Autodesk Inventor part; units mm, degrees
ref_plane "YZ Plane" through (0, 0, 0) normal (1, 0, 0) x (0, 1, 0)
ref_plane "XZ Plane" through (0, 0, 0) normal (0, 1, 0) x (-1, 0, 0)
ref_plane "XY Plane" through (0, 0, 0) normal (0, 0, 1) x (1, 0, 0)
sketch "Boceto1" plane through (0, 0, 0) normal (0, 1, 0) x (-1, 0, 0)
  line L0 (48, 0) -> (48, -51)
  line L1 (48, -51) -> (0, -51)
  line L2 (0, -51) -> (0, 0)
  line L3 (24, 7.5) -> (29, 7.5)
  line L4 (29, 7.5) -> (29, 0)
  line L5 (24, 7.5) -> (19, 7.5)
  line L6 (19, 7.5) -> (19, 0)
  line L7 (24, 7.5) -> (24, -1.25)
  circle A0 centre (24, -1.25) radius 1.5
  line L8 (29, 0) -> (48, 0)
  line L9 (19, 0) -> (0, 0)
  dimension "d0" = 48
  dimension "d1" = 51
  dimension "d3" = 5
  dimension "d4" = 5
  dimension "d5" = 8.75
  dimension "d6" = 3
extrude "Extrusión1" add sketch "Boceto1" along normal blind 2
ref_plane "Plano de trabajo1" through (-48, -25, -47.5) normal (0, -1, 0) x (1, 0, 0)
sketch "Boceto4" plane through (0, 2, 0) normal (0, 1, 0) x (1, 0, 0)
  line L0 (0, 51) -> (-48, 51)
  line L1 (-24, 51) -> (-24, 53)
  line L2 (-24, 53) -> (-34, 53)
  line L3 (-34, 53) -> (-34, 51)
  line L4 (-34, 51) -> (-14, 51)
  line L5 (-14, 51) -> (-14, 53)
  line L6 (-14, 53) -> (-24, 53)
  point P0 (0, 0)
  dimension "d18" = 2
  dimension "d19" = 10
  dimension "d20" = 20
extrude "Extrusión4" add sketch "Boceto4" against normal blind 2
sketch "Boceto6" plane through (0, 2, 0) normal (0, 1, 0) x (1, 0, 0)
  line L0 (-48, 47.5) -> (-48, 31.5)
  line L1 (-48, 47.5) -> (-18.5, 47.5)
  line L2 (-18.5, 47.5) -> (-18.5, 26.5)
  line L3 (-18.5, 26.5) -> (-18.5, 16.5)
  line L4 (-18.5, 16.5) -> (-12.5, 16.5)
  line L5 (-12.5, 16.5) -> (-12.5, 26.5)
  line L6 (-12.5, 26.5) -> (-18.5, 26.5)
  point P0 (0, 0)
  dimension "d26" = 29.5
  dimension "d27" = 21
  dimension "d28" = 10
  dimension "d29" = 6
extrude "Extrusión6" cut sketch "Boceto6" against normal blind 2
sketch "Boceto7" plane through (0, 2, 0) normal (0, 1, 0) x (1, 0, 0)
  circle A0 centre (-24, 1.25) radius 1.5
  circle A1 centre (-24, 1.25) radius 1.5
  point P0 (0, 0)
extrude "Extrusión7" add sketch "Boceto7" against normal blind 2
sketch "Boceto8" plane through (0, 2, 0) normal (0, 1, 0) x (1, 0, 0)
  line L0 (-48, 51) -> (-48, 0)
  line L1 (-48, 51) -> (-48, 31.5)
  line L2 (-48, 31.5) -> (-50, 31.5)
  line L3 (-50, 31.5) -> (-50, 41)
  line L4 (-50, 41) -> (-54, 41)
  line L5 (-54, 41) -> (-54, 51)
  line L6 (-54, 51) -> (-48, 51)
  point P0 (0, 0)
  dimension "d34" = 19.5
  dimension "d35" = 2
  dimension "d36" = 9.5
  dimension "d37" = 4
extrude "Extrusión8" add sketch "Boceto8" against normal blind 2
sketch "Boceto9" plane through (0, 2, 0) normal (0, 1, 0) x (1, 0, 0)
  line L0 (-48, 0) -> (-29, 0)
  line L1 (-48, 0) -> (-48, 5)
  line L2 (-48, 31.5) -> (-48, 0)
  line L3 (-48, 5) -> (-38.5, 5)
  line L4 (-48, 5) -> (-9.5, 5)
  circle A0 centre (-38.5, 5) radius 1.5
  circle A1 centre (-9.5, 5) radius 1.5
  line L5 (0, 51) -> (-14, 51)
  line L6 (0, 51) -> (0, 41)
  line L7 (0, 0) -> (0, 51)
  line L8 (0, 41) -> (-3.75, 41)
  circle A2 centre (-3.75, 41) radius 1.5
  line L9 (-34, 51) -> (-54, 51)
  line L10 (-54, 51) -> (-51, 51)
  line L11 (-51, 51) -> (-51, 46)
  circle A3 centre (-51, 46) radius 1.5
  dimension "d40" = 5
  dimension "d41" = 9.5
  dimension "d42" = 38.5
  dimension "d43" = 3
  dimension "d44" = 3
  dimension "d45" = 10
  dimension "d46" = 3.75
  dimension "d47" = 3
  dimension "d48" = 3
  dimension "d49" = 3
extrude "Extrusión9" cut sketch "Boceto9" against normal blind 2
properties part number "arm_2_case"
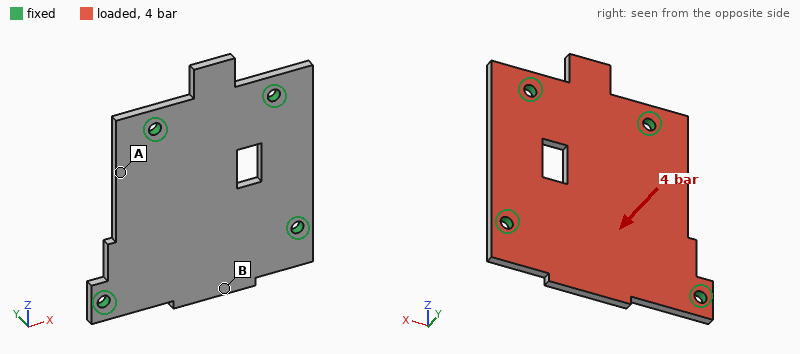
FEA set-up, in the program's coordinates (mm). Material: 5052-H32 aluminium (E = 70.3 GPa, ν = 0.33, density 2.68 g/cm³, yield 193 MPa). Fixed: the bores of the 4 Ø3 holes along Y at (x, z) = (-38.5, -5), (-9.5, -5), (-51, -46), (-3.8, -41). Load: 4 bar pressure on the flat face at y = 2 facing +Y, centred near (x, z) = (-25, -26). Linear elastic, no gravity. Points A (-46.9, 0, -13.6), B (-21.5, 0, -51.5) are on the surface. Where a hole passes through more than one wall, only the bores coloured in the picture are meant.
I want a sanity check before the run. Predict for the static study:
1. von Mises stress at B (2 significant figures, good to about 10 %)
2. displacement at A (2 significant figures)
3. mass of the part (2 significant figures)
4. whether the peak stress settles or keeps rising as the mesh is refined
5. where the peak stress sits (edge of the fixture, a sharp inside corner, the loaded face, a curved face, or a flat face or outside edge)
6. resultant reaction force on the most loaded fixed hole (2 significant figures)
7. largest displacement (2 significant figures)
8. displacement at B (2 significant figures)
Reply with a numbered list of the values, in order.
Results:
1. 50 MPa
2. 0.037 mm
3. 14 g
4. keeps rising
5. edge of the fixture
6. 300 N
7. 0.14 mm
8. 0.13 mm
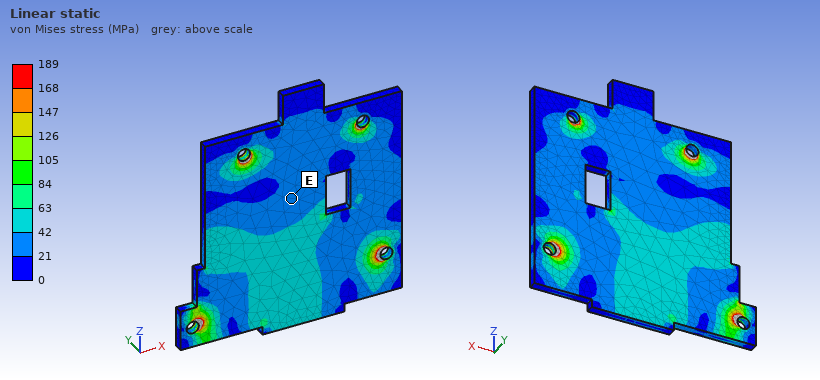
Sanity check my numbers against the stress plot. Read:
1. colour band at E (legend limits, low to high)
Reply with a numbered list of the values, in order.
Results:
1. 21 to 42 MPa
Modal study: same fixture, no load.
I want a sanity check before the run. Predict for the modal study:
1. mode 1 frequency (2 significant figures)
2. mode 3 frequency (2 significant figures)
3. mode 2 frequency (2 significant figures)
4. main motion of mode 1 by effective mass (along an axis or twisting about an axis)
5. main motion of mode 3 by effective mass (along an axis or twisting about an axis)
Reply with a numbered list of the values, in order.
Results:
1. 4300 Hz
2. 7700 Hz
3. 5800 Hz
4. along Y
5. twisting about Z
